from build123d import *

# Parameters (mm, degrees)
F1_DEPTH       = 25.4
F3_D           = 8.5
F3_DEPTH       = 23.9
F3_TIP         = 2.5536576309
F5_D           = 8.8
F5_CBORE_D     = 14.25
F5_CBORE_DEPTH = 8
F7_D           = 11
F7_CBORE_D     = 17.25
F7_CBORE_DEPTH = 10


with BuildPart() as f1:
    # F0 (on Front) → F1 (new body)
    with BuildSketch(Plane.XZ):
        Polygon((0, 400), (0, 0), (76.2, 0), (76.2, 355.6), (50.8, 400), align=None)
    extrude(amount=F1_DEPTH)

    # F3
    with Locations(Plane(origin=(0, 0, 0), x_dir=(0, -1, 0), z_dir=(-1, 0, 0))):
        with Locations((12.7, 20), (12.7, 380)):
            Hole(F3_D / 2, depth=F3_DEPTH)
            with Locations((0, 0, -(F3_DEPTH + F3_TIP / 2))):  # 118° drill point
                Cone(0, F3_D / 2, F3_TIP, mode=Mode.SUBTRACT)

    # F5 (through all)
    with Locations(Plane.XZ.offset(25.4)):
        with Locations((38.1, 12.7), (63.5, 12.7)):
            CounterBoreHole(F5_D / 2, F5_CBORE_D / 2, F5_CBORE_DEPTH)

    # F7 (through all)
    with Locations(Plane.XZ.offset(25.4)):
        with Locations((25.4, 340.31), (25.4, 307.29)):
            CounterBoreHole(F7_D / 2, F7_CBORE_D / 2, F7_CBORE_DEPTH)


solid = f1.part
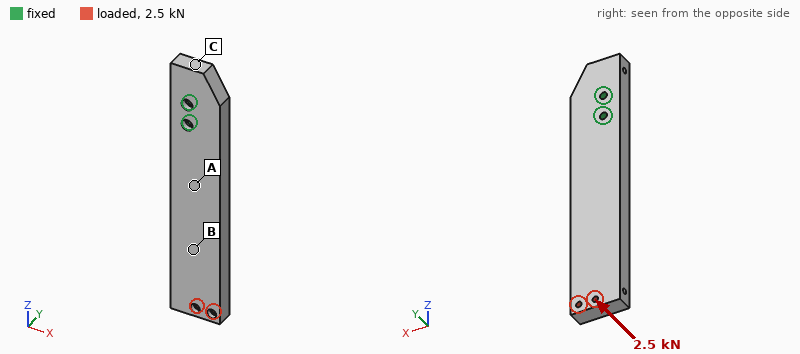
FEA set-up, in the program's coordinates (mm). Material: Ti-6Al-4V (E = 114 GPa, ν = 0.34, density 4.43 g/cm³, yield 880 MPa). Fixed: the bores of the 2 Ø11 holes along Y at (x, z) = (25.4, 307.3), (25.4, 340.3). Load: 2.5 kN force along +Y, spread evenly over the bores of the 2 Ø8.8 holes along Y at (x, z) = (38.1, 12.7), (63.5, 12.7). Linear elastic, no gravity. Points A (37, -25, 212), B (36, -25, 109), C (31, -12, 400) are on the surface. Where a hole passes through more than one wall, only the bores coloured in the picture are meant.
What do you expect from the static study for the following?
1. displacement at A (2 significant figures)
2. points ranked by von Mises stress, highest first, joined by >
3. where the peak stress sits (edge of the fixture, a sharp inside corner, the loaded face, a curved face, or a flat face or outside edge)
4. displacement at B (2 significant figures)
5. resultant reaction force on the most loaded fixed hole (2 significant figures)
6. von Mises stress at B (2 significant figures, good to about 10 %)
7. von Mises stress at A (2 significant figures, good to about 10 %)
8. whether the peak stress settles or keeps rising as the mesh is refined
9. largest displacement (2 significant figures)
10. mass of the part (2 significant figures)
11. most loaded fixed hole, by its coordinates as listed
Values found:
0.36 mm
A > B > C
edge of the fixture
1.2 mm
17 kN
30 MPa
61 MPa
keeps rising
2.3 mm
3.3 kg
(25.4, 307.3)
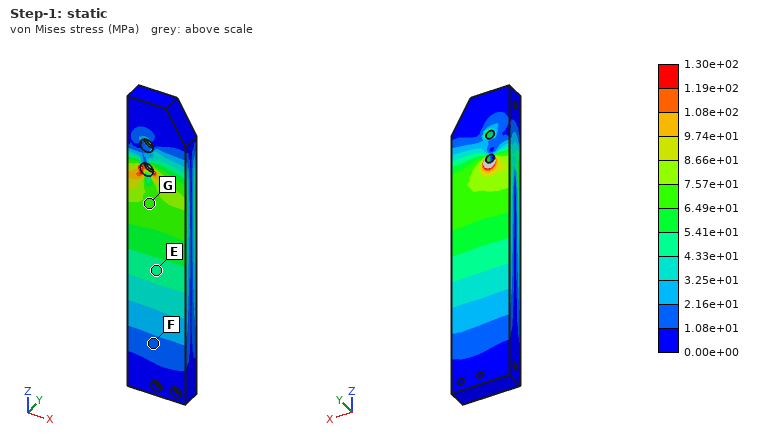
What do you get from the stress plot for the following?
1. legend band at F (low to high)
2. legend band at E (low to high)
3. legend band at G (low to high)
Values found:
1.08e+01 to 2.16e+01 MPa
4.33e+01 to 5.41e+01 MPa
6.49e+01 to 7.57e+01 MPa
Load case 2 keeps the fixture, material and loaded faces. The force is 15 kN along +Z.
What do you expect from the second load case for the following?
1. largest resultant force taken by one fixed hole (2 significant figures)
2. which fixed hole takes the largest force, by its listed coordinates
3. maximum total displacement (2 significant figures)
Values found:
13 kN
(25.4, 307.3)
0.30 mm
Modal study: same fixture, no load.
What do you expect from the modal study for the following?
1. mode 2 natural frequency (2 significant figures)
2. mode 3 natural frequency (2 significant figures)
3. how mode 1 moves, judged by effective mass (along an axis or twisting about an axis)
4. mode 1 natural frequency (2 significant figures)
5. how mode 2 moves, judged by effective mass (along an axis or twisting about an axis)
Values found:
470 Hz
1200 Hz
along Y
200 Hz
along X
